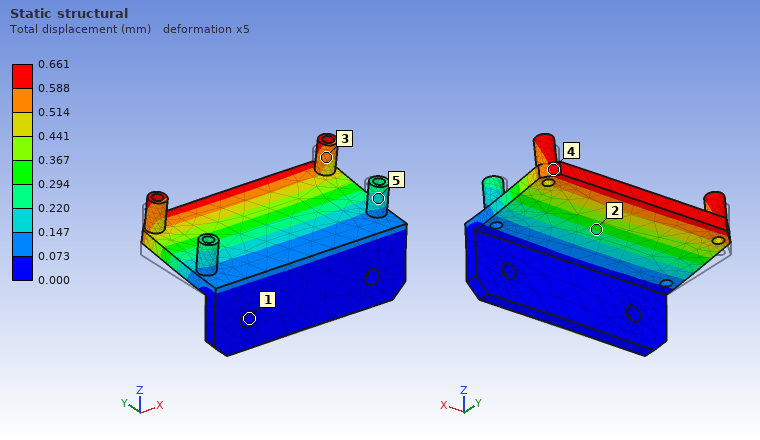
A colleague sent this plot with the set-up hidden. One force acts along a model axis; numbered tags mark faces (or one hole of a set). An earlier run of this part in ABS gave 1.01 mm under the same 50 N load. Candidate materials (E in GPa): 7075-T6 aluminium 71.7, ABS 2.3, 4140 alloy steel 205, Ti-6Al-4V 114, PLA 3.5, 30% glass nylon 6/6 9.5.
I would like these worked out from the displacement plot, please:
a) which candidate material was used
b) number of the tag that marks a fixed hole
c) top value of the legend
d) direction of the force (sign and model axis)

PLA
1
0.661 mm
+Z
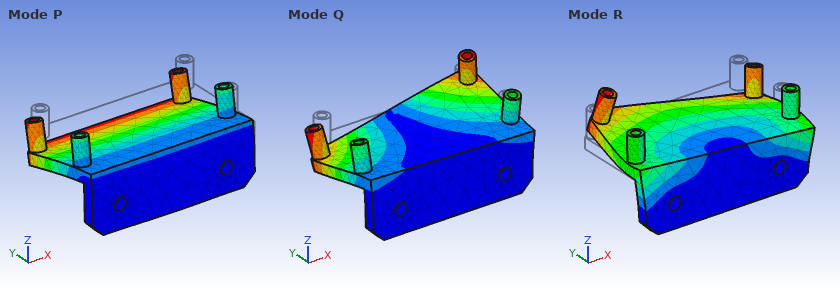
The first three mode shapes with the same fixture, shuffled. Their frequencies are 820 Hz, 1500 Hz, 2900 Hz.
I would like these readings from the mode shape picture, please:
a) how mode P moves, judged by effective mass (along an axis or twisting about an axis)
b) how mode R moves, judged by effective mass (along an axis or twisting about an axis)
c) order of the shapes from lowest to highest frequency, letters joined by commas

along Z
along X
P, Q, R
